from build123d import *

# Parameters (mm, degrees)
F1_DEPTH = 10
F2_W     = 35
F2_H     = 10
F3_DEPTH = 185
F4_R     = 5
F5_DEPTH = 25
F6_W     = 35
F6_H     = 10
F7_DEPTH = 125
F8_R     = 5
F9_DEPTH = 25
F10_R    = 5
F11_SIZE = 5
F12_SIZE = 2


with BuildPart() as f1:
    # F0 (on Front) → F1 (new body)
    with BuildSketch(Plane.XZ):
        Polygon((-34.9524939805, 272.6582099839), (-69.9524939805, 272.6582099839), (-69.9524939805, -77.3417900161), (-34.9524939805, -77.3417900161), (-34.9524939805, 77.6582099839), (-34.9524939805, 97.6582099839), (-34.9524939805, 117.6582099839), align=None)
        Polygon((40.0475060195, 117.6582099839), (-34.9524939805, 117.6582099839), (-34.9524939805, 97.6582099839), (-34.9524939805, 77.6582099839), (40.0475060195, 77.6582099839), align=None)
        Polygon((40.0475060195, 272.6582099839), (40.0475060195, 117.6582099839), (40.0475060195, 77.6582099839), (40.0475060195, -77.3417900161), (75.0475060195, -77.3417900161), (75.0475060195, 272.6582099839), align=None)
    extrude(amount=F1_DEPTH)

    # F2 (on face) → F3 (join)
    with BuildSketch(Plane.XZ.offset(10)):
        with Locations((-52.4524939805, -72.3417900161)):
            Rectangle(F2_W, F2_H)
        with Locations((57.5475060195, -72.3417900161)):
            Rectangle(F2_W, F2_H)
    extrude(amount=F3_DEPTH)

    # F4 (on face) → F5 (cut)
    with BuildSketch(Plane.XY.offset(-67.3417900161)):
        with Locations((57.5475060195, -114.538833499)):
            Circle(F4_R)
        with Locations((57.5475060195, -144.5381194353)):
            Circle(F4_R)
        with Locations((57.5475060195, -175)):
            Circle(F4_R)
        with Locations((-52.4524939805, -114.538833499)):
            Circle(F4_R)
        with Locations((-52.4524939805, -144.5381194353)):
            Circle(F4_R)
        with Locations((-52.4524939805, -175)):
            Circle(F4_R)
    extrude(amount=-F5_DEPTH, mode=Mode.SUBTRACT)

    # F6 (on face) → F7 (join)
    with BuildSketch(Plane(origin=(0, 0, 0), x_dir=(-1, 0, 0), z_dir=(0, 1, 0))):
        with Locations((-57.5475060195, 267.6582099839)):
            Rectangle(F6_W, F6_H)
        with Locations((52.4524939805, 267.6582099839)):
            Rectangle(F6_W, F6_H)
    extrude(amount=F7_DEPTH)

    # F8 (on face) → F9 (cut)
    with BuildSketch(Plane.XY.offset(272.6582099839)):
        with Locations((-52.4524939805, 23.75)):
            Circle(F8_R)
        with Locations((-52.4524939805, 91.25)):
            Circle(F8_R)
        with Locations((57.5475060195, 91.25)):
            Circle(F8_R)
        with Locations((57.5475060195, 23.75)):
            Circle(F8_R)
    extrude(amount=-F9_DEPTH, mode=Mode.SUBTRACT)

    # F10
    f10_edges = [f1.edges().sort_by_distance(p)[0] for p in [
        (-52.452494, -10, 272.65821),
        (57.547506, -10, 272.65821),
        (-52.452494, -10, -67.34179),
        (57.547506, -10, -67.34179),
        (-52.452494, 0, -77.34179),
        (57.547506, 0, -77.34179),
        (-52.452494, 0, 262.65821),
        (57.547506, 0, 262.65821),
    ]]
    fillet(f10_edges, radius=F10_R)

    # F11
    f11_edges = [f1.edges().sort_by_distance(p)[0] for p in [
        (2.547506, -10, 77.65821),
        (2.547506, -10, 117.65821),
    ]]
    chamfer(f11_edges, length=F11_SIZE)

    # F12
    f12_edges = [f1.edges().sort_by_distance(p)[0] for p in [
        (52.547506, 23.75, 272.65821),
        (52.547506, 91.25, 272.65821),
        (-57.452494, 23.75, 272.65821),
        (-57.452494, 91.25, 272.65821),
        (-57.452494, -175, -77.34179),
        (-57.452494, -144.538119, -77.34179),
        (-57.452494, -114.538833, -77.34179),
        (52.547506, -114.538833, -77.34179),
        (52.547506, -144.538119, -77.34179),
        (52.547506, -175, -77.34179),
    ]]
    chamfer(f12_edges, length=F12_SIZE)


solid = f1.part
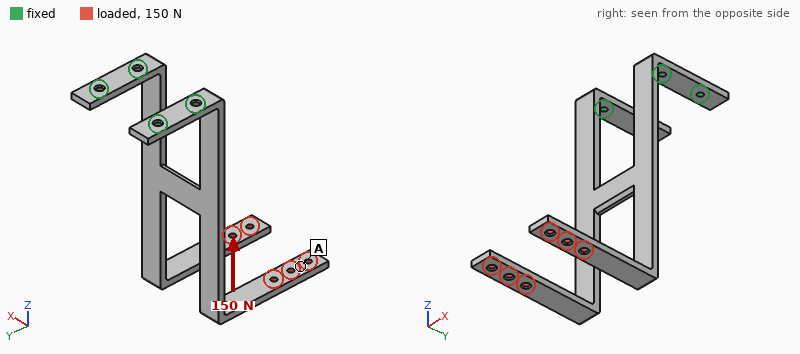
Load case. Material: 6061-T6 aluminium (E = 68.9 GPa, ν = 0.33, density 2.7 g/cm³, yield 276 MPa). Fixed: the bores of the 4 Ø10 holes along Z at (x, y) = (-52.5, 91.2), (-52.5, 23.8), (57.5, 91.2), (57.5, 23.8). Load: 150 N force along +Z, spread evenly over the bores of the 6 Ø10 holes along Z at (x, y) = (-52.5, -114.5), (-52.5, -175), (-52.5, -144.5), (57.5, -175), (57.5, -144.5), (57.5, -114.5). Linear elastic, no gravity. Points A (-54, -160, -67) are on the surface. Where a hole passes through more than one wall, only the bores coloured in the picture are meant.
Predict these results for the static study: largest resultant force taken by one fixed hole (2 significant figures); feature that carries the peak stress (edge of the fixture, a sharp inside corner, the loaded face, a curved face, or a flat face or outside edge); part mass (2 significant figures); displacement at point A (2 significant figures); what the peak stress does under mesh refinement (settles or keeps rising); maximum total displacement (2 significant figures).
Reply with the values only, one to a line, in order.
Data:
100 N
edge of the fixture
1.3 kg
4.6 mm
keeps rising
5.3 mm
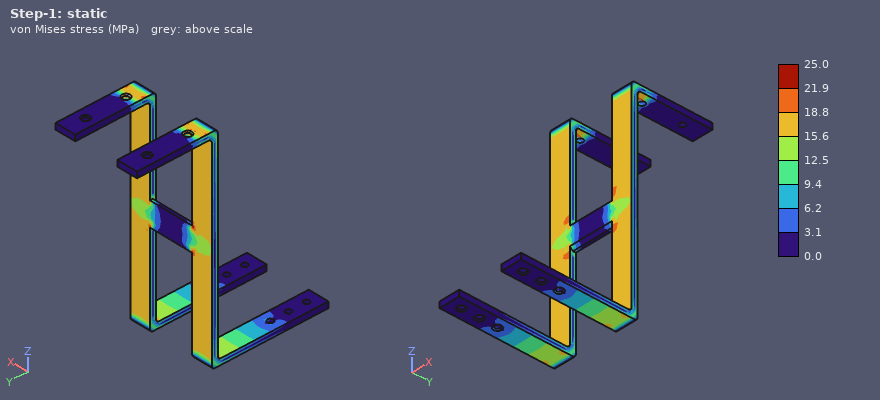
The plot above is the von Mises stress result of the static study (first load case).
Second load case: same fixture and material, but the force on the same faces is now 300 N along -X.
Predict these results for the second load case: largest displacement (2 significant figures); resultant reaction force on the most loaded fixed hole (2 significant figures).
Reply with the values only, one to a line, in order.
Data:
4.8 mm
830 N
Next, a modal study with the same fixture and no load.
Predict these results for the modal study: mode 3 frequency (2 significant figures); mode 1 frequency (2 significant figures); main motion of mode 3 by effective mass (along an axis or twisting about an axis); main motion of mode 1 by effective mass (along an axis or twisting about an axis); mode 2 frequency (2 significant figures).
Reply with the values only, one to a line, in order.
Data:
110 Hz
34 Hz
along X
along Y
71 Hz
